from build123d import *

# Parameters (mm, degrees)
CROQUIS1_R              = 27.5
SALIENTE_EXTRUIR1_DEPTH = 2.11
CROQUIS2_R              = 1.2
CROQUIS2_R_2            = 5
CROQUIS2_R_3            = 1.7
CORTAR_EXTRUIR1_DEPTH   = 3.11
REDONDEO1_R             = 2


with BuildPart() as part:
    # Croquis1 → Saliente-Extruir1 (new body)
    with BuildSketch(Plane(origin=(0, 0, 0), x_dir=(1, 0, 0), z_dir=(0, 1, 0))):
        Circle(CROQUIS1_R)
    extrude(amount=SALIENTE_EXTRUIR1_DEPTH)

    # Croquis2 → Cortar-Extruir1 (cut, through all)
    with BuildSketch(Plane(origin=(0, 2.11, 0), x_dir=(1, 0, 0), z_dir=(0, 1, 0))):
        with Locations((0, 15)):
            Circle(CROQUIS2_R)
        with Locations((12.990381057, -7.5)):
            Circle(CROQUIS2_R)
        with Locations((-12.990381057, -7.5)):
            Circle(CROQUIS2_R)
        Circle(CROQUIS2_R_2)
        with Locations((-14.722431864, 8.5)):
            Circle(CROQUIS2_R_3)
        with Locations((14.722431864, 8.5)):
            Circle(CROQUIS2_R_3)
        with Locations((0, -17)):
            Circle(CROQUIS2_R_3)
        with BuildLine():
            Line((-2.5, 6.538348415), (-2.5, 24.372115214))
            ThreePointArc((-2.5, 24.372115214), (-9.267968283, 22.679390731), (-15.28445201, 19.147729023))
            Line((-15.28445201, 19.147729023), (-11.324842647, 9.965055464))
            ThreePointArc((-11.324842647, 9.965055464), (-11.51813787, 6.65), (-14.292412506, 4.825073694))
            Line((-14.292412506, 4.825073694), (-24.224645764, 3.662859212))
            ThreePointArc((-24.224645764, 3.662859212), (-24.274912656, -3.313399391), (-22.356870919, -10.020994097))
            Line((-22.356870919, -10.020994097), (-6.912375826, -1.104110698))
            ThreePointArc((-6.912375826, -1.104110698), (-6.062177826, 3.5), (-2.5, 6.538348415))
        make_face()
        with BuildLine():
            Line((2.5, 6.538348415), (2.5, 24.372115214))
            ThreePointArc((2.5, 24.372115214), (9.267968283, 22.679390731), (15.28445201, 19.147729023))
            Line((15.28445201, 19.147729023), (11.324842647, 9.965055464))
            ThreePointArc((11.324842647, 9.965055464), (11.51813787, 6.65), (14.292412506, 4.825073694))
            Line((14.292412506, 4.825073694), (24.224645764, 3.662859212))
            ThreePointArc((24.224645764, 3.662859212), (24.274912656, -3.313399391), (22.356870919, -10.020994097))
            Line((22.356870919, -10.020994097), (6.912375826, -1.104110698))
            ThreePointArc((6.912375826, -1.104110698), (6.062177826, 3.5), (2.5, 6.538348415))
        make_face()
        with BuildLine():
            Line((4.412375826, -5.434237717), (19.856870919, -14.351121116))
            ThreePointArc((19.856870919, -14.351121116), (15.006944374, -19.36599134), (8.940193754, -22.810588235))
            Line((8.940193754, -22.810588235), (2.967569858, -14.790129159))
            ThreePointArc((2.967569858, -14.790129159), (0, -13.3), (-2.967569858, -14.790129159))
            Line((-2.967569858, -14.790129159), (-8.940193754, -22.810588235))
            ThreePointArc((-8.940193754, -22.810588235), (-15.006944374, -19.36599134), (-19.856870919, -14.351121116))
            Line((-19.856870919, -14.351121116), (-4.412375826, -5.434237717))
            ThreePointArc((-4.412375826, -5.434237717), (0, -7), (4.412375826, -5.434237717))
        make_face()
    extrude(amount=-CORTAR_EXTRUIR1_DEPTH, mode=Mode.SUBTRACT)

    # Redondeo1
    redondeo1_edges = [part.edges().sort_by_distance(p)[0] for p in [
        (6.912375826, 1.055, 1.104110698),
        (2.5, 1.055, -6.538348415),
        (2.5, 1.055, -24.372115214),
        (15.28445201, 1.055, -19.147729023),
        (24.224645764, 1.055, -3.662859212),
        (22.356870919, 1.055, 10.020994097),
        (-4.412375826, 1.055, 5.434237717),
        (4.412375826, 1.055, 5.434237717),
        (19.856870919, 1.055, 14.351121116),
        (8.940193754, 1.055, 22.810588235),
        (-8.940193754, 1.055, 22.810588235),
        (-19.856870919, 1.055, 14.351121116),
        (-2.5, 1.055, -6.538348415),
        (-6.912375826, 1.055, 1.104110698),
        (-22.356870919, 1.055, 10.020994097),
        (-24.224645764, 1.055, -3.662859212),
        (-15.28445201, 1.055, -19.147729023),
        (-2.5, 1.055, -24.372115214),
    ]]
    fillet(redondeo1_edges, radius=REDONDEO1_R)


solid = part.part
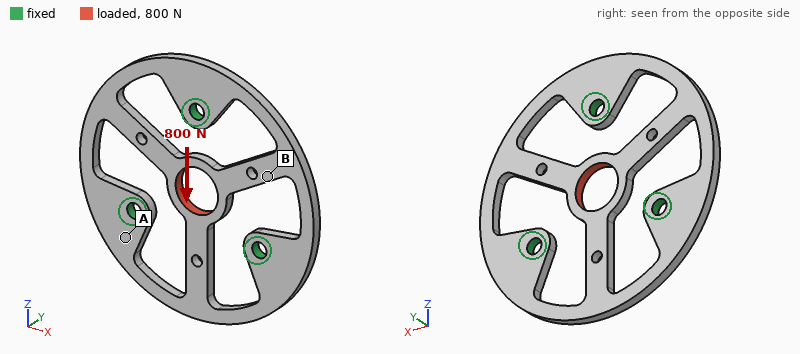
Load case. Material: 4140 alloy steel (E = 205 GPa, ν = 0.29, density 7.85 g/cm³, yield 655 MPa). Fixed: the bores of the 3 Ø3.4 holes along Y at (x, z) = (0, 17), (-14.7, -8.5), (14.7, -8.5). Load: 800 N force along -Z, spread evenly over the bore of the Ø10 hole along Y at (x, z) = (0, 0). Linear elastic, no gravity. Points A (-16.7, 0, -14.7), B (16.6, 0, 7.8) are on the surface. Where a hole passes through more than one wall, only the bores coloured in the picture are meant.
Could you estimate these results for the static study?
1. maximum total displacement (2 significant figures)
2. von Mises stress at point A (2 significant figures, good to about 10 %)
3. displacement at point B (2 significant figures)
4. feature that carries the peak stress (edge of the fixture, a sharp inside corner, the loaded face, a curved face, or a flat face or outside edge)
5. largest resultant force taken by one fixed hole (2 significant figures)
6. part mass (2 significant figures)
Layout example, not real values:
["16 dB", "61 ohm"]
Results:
["73 µm", "48 MPa", "29 µm", "a curved face", "460 N", "19 g"]
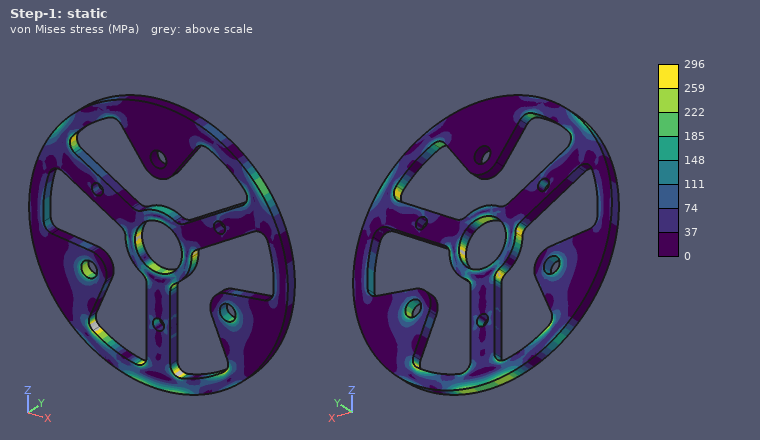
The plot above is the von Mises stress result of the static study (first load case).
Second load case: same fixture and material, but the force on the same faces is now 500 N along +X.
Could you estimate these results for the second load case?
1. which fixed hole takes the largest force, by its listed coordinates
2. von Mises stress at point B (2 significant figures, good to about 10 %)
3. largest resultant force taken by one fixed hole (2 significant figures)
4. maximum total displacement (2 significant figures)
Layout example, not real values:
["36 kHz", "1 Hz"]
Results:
["(0, 17)", "38 MPa", "330 N", "44 µm"]
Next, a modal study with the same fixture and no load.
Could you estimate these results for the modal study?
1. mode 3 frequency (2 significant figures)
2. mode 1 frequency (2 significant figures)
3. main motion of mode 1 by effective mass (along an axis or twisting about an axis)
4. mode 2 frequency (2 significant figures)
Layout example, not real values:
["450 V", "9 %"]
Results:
["3700 Hz", "2700 Hz", "along Y", "3700 Hz"]
